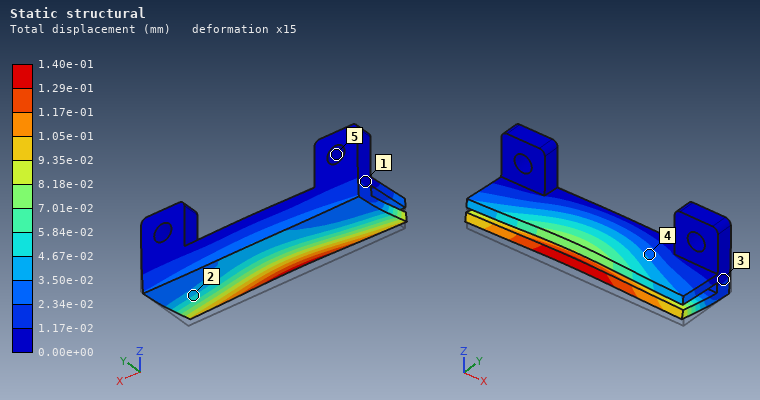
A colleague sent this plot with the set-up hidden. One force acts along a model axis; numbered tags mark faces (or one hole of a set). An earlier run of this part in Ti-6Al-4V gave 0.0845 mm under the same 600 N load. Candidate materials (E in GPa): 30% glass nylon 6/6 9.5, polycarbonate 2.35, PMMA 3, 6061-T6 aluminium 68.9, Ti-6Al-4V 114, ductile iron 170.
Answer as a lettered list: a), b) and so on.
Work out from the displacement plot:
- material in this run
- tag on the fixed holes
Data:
a) 6061-T6 aluminium
b) 5
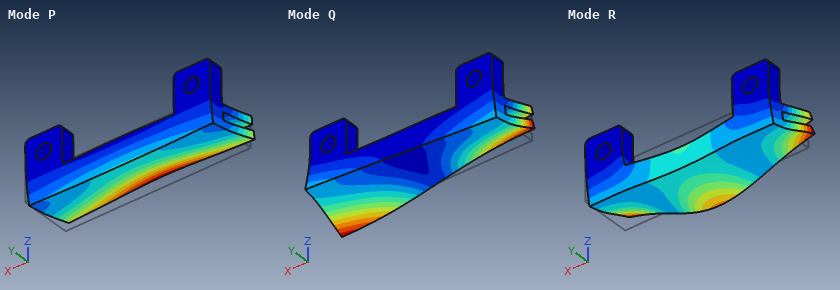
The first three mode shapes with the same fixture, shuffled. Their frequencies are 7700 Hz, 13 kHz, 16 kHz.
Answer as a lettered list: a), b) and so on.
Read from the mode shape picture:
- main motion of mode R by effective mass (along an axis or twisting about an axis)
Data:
a) along Y
